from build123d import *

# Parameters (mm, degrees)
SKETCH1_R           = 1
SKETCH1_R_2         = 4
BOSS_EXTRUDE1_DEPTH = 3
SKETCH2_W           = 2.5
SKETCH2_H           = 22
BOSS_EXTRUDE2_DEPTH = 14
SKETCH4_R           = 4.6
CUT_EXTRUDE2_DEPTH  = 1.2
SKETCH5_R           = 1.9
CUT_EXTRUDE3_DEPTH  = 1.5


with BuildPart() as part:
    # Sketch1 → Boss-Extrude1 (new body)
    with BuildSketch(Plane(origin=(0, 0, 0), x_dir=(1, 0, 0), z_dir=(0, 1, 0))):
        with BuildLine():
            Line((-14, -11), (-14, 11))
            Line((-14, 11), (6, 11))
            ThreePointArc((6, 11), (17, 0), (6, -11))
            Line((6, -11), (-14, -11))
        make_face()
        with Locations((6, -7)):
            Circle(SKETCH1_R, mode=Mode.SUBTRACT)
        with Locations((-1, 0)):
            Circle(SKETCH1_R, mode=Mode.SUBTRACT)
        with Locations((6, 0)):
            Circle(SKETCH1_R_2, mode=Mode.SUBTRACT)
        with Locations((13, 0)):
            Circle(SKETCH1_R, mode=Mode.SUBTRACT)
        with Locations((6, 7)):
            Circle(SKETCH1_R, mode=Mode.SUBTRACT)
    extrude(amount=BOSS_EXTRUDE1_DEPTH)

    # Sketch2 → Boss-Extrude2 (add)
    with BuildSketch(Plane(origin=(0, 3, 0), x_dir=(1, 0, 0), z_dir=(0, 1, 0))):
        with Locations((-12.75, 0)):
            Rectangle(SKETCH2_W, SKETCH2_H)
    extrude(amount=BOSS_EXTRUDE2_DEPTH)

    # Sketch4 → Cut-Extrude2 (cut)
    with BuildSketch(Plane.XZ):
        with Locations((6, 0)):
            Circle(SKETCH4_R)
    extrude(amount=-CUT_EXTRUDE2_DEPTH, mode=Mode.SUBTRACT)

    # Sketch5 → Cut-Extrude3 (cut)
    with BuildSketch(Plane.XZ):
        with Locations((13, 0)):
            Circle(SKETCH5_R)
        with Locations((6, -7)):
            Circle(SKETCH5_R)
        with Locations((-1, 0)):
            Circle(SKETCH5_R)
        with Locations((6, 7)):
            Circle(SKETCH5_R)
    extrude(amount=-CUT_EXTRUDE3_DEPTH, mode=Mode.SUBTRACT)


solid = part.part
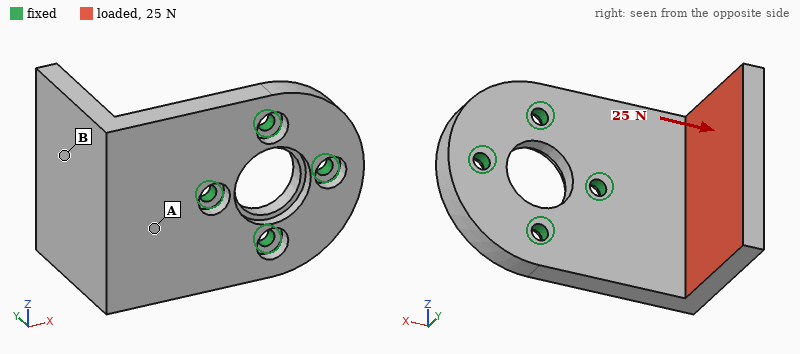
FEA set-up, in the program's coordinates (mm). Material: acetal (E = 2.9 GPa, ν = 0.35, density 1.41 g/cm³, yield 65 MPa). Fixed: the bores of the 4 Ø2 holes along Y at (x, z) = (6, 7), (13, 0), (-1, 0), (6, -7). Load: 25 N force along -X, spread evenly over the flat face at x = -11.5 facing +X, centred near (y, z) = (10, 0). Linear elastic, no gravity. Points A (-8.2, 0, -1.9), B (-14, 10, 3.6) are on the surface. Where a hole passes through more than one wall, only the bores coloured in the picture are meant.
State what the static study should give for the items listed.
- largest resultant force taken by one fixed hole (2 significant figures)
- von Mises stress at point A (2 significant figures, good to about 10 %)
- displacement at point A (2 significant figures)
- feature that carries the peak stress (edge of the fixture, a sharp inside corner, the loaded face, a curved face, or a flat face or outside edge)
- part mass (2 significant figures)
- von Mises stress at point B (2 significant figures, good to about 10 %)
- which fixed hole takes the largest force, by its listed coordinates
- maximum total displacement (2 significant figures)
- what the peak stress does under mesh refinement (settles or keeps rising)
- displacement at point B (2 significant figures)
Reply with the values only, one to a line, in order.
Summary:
39 N
5.2 MPa
0.076 mm
edge of the fixture
3.4 g
1.7 MPa
(-1, 0)
0.47 mm
keeps rising
0.29 mm
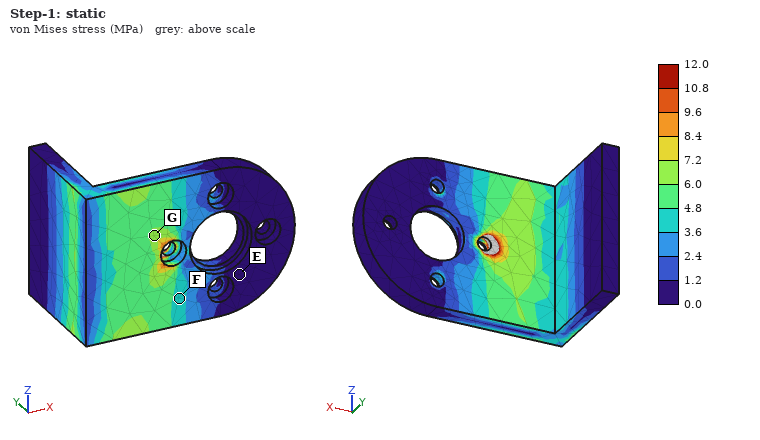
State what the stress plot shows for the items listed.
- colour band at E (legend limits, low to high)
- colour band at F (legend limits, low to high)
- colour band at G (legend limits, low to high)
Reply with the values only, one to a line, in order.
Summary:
0.0 to 1.2 MPa
3.6 to 4.8 MPa
6.0 to 7.2 MPa
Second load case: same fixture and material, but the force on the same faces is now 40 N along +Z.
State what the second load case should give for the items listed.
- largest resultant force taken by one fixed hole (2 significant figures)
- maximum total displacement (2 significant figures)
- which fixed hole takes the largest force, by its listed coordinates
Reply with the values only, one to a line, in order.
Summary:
52 N
0.49 mm
(-1, 0)
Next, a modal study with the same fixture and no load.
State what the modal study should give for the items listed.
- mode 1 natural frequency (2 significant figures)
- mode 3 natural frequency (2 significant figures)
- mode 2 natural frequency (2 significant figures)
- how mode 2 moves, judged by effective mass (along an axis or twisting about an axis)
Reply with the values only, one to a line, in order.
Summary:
1100 Hz
2600 Hz
1400 Hz
along Z
